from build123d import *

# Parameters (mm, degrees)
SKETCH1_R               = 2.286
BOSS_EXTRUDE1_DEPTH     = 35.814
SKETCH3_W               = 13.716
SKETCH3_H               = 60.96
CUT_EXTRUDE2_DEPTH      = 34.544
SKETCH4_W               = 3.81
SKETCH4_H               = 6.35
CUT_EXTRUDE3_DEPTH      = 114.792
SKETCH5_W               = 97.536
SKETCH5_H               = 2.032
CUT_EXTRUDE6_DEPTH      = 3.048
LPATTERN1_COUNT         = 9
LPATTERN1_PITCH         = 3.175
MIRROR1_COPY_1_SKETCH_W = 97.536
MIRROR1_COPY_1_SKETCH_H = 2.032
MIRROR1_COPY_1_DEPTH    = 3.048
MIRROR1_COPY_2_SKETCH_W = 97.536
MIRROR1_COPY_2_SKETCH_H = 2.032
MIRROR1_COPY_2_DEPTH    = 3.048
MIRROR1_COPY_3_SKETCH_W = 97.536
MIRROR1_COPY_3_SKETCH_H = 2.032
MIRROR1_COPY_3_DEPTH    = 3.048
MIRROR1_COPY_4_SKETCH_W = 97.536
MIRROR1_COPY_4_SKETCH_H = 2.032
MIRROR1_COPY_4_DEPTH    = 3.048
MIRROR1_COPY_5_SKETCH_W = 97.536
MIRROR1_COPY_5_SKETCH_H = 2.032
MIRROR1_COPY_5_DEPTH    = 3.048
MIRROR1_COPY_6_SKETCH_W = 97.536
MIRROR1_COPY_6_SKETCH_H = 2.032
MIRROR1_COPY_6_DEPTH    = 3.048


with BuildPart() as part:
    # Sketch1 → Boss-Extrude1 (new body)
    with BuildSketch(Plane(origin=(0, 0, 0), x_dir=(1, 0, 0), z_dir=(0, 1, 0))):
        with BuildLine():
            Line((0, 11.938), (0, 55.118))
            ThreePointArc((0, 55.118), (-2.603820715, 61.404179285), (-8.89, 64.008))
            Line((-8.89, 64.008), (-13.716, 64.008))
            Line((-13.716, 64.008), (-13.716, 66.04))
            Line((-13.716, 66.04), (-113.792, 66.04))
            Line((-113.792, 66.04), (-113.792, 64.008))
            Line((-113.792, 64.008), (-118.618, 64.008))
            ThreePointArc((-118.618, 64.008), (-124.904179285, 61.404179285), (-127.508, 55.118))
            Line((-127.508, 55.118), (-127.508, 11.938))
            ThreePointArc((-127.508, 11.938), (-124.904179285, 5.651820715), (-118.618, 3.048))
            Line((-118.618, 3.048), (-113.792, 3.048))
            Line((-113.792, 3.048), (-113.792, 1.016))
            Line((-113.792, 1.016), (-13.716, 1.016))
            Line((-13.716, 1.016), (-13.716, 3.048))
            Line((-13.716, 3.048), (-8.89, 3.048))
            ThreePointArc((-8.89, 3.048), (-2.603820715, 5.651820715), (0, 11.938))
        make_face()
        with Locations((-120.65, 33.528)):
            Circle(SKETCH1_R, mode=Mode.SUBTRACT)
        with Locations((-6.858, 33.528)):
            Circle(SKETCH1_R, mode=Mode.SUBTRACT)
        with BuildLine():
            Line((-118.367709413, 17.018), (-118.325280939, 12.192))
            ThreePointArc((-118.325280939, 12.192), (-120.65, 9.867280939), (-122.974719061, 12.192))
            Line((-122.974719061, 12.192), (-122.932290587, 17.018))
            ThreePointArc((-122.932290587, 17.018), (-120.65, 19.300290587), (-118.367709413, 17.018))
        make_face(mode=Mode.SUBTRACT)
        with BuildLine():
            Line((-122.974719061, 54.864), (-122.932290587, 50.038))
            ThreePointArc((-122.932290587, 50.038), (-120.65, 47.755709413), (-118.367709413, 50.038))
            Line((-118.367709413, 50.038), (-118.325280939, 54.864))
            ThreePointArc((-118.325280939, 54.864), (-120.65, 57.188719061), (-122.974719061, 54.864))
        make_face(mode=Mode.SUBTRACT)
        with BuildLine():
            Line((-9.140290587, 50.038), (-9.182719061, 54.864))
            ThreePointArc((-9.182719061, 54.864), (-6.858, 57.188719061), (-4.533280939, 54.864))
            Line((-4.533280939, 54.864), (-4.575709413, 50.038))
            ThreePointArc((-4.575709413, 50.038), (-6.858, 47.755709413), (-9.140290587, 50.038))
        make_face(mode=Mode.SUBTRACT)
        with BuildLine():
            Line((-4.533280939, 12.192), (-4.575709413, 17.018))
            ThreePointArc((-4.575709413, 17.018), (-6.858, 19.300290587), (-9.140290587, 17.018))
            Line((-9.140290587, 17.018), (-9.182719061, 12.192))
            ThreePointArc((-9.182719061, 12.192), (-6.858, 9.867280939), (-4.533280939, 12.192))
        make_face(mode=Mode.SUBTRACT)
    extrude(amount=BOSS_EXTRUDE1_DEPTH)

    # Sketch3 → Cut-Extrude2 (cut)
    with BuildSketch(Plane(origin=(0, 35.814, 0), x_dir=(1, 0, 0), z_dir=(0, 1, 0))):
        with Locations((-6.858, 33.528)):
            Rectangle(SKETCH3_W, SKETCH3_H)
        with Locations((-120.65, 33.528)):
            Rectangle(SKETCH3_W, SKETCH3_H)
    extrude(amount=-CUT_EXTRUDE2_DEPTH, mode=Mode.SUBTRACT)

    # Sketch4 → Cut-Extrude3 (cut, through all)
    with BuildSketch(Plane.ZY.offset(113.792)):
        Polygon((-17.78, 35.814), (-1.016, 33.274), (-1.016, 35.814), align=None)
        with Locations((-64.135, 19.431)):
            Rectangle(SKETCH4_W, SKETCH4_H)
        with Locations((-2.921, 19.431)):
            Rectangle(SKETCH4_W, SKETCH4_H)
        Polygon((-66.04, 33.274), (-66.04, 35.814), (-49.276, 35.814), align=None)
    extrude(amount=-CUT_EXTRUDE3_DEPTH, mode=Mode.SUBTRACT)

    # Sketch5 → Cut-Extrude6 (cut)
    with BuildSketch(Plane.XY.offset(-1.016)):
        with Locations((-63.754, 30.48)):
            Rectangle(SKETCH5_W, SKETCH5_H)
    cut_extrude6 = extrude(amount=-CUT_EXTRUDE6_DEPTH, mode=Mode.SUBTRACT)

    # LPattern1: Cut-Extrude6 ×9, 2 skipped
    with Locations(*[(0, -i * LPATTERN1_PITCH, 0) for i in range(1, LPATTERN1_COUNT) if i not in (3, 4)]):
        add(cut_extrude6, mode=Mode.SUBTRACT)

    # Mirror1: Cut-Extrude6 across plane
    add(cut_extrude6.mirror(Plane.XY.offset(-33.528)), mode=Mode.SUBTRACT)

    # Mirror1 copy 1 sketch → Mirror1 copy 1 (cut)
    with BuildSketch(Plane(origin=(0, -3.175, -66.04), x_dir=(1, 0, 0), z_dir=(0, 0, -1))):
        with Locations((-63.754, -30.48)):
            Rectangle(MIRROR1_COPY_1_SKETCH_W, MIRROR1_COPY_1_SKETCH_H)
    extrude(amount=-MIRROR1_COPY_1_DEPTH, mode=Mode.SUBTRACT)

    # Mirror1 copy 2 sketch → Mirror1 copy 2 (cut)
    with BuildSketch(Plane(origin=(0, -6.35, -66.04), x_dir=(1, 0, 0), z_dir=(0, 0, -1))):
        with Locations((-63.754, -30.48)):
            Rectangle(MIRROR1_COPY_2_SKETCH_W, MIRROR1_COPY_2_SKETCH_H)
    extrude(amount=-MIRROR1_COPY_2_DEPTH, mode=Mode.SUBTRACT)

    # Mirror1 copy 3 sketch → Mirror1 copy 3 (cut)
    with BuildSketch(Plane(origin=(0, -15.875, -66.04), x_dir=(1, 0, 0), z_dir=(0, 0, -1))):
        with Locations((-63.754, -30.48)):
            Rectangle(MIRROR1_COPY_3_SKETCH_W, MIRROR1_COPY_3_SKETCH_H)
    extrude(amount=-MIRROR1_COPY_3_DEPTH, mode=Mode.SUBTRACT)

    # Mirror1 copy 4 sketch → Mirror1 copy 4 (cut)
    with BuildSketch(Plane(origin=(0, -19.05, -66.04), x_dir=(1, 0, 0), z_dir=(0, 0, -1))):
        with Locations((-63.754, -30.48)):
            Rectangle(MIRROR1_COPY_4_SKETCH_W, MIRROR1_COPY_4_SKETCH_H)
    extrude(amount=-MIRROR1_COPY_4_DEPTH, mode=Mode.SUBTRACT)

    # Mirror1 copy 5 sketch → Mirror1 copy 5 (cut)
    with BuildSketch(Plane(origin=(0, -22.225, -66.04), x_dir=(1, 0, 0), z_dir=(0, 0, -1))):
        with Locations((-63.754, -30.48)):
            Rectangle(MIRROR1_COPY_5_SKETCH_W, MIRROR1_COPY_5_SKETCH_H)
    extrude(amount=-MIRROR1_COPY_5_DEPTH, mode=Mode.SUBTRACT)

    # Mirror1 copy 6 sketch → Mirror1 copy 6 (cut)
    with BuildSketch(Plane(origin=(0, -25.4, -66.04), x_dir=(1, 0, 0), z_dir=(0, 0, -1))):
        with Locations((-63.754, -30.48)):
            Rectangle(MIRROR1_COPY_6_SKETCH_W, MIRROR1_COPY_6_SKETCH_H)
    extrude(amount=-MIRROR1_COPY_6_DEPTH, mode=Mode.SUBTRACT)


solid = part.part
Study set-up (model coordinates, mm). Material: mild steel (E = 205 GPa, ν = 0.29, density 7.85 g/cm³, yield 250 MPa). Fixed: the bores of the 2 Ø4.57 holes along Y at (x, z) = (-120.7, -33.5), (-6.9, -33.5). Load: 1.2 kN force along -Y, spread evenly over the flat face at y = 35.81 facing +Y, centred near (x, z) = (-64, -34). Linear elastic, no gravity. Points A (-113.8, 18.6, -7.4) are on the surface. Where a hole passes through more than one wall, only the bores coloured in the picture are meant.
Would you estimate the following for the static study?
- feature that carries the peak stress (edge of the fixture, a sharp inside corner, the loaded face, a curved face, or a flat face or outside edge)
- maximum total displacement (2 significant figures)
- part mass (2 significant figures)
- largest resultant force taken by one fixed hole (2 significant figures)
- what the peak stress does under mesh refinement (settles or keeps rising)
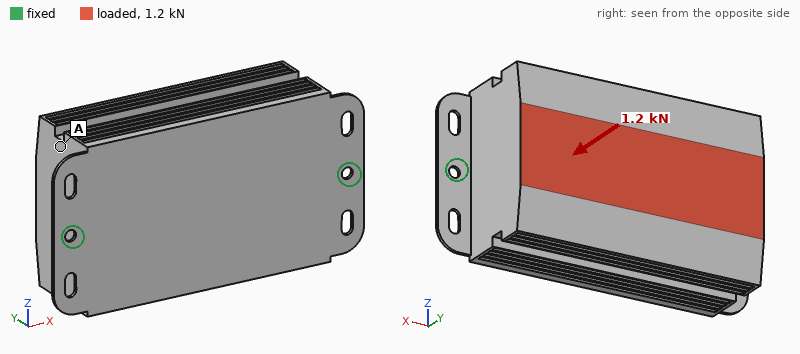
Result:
edge of the fixture
25 µm
1.7 kg
690 N
keeps rising
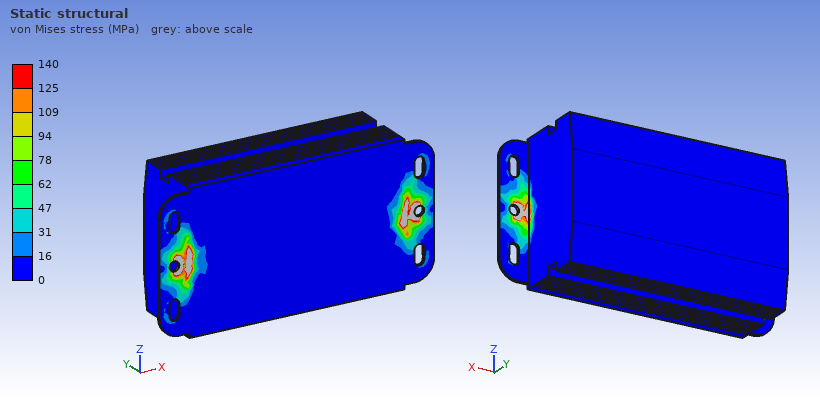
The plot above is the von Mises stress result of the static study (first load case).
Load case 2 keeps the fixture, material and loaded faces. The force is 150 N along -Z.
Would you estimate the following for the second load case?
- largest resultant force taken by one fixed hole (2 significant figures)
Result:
75 N
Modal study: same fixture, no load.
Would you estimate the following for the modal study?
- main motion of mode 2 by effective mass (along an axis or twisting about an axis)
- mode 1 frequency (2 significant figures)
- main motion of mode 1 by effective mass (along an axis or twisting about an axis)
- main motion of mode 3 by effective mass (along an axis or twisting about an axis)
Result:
along Y
140 Hz
along Z
along X
